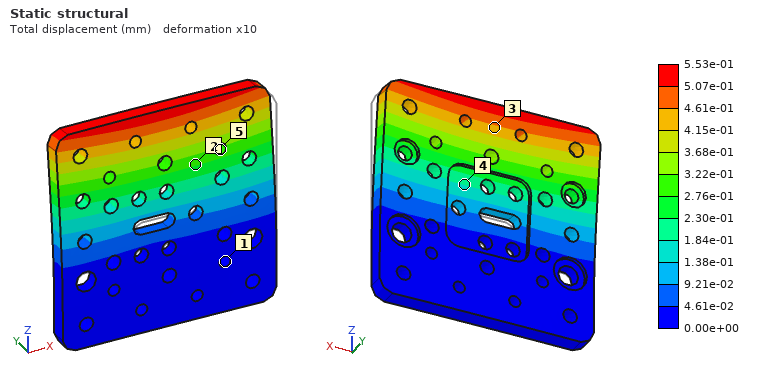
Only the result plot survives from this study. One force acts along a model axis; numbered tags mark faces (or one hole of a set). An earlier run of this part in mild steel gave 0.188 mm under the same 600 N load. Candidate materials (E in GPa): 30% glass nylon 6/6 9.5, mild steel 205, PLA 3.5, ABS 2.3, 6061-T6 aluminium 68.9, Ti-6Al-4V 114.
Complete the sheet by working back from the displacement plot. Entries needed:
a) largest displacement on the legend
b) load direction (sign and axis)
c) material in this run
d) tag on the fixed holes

5.53e-01 mm
+Y
6061-T6 aluminium
1
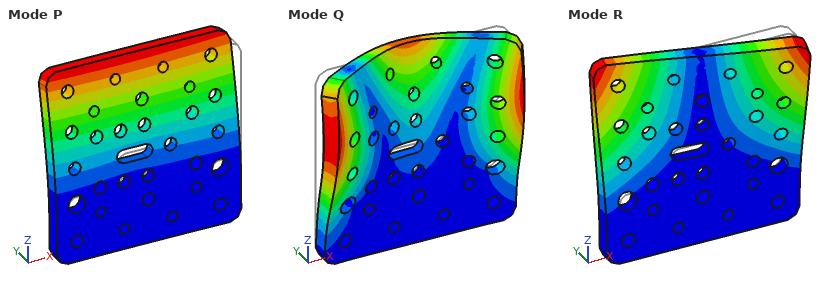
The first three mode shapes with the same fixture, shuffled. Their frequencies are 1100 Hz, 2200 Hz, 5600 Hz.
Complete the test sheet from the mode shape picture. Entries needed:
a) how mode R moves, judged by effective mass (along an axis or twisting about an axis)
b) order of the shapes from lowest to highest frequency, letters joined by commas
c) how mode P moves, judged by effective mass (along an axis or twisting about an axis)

twisting about Z
P, R, Q
along Y
